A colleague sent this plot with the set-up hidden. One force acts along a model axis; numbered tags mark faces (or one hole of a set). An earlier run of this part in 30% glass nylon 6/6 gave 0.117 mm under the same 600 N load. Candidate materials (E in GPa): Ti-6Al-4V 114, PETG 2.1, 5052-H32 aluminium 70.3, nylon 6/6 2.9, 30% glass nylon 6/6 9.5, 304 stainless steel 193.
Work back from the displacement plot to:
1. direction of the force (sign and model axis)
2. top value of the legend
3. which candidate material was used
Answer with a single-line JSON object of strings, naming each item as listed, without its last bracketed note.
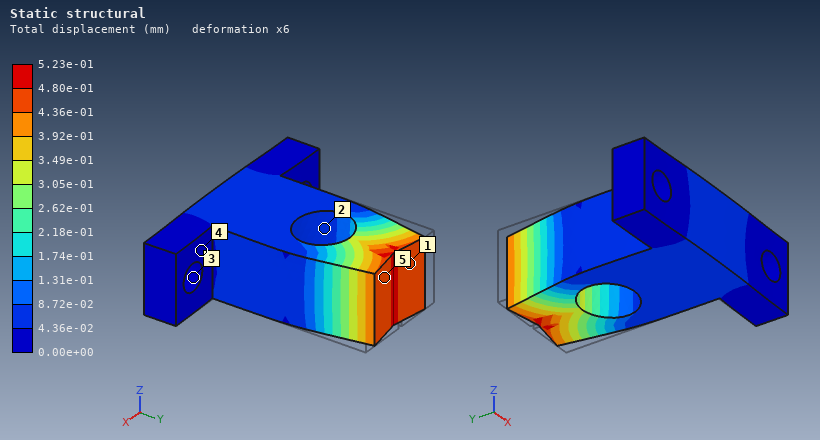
{"direction of the force": "-Y", "top value of the legend": "5.23e-01 mm", "which candidate material was used": "PETG"}
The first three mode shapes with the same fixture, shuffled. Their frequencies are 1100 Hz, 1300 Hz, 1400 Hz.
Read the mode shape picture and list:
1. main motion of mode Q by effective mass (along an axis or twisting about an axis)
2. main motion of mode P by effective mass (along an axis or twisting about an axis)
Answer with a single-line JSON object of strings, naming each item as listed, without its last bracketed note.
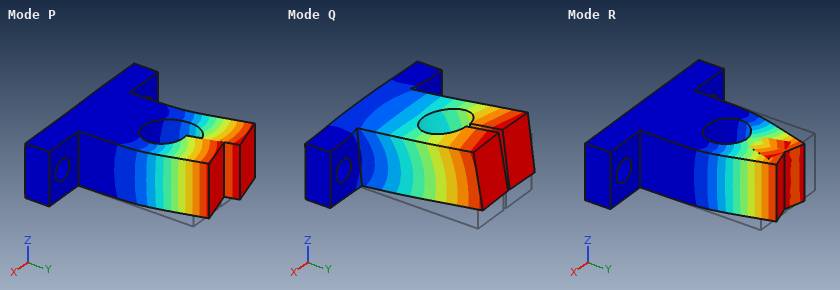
{"main motion of mode Q by effective mass": "along Z", "main motion of mode P by effective mass": "along X"}
